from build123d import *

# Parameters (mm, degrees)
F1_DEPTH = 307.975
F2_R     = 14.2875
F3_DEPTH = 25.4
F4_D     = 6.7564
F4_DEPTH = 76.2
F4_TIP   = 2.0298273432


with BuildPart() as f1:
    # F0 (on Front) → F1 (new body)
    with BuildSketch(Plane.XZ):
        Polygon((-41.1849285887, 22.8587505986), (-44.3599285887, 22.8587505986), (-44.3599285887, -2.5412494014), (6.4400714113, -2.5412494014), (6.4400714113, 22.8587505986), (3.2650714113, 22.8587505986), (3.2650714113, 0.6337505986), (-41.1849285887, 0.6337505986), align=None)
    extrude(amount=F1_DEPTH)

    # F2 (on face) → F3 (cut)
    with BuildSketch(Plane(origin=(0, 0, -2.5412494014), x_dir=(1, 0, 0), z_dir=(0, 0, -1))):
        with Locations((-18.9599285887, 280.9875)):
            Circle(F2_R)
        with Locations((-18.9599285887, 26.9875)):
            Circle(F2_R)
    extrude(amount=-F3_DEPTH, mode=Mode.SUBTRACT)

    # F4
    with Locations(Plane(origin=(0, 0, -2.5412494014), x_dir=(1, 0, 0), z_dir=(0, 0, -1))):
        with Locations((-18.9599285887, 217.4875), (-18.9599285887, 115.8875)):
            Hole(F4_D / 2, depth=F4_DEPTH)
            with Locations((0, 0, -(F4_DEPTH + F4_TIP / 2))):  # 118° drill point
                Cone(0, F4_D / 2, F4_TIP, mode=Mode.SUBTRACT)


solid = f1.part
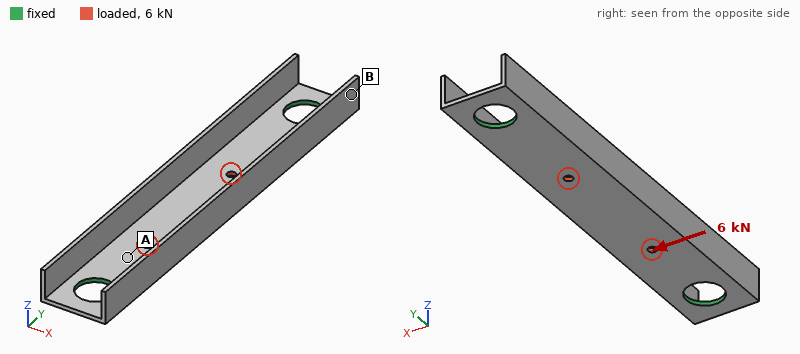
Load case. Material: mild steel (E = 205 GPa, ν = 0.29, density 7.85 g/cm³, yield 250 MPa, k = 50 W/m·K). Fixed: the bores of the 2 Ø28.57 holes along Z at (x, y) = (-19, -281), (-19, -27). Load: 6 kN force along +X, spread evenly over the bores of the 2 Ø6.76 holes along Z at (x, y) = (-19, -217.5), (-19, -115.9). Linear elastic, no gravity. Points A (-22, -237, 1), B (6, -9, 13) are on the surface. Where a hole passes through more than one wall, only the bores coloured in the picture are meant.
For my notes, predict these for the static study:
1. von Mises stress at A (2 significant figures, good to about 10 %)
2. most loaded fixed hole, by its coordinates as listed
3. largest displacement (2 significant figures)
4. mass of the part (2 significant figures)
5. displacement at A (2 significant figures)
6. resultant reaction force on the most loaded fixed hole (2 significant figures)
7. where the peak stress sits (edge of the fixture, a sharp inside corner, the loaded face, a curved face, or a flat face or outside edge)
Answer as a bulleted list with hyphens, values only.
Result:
- 58 MPa
- (-19, -281)
- 0.10 mm
- 700 g
- 0.022 mm
- 3.4 kN
- edge of the fixture
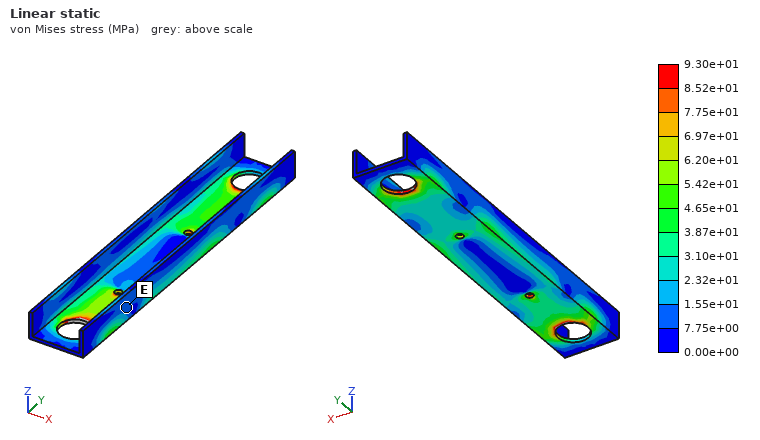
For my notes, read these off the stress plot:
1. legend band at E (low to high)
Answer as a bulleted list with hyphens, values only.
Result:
- 7.75e+00 to 1.55e+01 MPa
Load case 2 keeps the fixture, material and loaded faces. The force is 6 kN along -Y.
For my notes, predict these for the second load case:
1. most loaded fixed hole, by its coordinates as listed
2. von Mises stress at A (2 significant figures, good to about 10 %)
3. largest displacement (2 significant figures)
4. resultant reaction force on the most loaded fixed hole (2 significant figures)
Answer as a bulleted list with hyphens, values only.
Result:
- (-19, -281)
- 24 MPa
- 8.6 µm
- 3.3 kN
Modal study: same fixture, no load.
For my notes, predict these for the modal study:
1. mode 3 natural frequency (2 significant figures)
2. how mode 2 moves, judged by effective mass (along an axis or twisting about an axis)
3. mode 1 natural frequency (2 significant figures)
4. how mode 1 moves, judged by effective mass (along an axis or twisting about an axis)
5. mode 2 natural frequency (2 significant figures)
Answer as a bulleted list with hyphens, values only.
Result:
- 2200 Hz
- along Z
- 1200 Hz
- along X
- 1200 Hz
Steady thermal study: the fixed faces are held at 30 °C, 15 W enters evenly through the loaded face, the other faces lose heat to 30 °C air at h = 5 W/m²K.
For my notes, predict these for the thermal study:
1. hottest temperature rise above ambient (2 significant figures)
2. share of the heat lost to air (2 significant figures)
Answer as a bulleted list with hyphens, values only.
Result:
- 40 K
- 30 %
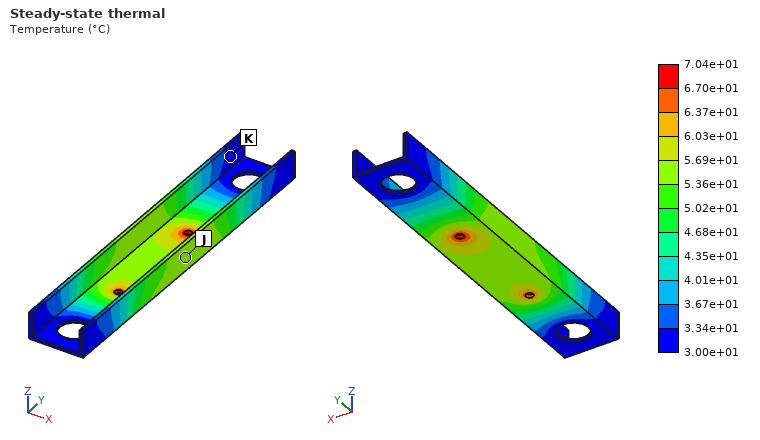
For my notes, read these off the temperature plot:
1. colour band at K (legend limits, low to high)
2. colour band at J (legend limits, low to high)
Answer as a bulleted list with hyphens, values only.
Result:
- 3.00e+01 to 3.34e+01 °C
- 5.36e+01 to 5.69e+01 °C
